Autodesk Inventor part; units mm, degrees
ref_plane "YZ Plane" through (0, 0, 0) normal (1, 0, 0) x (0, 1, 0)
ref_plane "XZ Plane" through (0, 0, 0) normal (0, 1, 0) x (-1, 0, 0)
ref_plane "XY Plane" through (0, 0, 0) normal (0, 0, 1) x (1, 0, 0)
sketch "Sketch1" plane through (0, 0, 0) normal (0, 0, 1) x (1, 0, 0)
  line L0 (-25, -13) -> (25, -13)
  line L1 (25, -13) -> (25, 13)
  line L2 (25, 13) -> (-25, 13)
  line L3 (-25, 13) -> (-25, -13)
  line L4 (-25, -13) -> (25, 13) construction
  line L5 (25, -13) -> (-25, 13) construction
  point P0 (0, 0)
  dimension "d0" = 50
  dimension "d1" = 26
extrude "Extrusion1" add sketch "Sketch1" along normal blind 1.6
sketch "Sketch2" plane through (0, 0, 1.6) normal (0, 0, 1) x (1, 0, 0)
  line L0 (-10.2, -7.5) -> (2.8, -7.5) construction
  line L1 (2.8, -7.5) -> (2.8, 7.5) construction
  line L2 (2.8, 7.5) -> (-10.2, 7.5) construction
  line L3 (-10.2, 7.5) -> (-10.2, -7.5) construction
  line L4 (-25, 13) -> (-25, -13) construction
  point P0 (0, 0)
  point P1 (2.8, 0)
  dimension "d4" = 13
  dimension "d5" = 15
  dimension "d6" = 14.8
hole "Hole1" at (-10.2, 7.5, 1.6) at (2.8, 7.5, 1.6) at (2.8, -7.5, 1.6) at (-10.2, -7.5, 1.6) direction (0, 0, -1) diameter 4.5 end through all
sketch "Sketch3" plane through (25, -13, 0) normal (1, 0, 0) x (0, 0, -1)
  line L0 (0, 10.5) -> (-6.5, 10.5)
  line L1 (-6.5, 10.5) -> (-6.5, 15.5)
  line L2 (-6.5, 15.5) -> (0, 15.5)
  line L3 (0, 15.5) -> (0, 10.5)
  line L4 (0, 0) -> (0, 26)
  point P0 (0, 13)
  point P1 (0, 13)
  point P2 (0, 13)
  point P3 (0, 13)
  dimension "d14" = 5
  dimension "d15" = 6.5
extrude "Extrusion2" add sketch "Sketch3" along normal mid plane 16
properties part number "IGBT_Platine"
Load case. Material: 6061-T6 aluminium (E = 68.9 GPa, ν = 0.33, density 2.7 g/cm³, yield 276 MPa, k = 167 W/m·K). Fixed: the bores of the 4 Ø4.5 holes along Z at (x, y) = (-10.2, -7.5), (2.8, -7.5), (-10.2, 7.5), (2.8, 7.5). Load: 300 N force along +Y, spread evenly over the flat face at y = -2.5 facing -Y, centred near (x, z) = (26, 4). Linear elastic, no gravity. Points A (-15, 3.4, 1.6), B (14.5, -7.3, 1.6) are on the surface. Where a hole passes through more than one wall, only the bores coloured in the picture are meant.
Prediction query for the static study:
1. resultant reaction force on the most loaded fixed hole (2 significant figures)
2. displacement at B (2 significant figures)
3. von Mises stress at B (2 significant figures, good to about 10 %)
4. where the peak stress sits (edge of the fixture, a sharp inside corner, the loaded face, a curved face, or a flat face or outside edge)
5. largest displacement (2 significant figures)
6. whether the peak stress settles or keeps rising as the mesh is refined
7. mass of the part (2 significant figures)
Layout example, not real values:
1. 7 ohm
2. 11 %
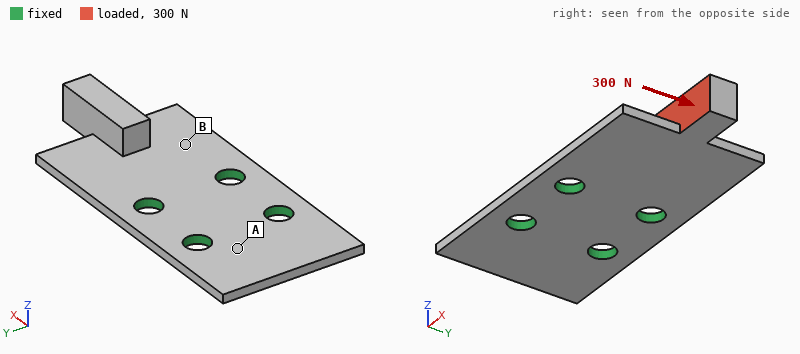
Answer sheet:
1. 380 N
2. 0.033 mm
3. 45 MPa
4. edge of the fixture
5. 0.10 mm
6. keeps rising
7. 6.6 g
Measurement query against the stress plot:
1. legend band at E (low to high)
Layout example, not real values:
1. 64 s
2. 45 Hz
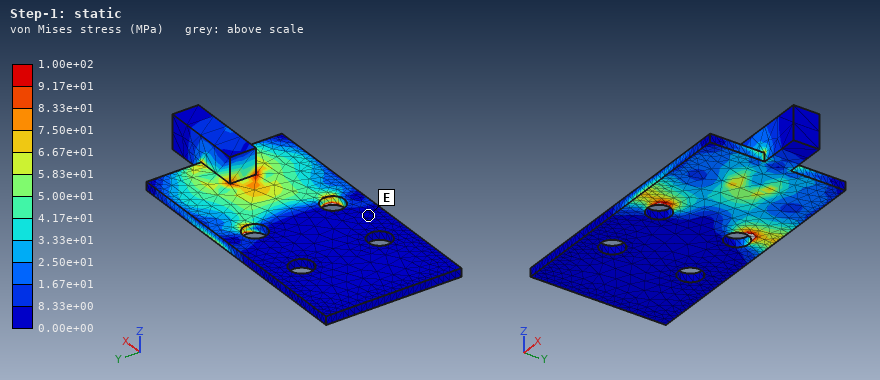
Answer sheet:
1. 0.00e+00 to 8.33e+00 MPa
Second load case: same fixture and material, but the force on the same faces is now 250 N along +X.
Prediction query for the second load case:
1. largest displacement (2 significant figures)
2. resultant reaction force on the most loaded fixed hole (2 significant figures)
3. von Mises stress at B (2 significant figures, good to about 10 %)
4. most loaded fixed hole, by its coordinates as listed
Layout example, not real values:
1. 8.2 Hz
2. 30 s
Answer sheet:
1. 0.37 mm
2. 150 N
3. 62 MPa
4. (2.8, -7.5)
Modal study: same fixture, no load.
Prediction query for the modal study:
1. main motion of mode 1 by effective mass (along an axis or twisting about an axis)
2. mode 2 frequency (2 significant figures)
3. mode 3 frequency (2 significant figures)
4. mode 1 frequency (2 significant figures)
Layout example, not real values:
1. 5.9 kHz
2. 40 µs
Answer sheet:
1. along Z
2. 6000 Hz
3. 7300 Hz
4. 1600 Hz
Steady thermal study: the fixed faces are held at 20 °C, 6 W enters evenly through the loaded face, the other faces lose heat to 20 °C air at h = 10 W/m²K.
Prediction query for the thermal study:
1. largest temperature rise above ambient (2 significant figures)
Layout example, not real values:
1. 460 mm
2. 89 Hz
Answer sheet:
1. 22 K
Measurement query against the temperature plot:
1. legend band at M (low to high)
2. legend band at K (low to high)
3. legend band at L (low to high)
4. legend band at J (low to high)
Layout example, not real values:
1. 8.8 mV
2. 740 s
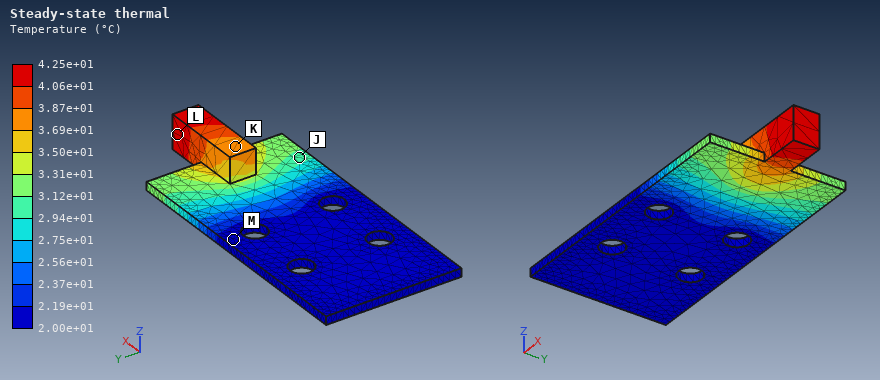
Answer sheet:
1. 2.00e+01 to 2.19e+01 °C
2. 3.69e+01 to 3.87e+01 °C
3. 4.06e+01 to 4.25e+01 °C
4. 2.94e+01 to 3.12e+01 °C
